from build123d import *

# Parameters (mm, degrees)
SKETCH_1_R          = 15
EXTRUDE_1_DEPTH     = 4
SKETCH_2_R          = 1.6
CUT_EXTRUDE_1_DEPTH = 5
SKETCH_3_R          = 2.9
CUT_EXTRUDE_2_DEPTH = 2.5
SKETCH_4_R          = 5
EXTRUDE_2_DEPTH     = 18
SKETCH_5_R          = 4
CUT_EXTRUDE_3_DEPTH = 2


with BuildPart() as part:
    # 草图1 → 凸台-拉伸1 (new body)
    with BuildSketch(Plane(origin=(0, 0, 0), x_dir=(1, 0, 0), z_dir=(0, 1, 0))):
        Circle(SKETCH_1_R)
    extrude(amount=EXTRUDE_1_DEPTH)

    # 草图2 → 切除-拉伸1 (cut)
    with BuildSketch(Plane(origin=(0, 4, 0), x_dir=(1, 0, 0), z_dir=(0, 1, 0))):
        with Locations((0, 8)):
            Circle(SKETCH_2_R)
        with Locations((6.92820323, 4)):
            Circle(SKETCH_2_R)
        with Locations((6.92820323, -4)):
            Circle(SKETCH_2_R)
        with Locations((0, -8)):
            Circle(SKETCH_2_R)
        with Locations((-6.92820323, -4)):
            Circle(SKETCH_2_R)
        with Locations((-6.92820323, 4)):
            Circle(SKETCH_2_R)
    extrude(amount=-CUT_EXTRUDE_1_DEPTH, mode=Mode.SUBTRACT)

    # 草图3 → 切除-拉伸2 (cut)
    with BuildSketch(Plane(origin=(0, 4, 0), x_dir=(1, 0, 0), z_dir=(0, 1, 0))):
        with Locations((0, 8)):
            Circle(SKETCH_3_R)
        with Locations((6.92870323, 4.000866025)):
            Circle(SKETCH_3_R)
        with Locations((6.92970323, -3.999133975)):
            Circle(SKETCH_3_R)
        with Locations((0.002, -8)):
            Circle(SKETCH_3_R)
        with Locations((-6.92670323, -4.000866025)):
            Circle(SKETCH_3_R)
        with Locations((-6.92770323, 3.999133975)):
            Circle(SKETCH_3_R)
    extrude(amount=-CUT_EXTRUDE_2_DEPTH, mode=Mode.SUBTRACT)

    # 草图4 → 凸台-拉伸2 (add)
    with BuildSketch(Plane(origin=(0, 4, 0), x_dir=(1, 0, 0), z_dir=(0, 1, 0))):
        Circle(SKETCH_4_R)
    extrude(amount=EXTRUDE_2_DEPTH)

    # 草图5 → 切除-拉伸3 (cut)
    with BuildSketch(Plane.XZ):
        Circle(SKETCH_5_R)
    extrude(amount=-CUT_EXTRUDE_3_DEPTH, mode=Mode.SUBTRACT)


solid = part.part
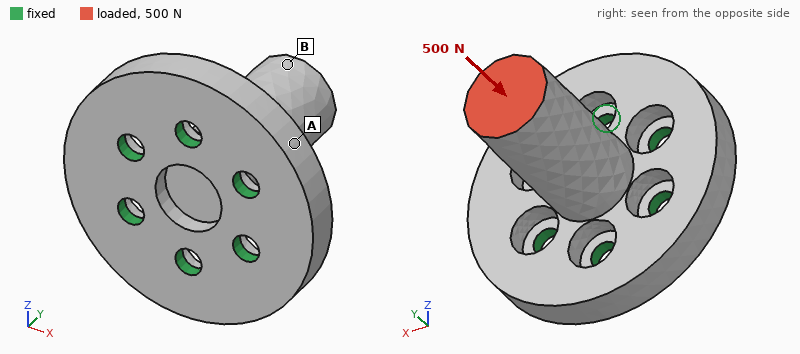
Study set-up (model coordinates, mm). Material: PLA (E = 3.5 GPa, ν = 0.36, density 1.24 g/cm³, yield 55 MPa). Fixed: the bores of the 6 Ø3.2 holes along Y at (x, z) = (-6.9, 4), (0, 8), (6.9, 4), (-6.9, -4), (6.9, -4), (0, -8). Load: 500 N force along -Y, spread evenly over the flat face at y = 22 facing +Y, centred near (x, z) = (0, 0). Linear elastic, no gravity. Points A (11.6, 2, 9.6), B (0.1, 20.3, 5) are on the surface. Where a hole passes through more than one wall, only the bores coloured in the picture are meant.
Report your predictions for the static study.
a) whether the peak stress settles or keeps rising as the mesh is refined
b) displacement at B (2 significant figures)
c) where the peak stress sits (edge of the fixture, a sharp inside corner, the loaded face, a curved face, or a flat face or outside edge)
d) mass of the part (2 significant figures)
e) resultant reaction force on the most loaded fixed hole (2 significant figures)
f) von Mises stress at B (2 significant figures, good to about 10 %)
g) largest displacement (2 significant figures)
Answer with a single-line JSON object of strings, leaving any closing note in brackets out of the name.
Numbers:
{"whether the peak stress settles or keeps rising as the mesh is refined": "keeps rising", "displacement at B": "56 µm", "where the peak stress sits": "edge of the fixture", "mass of the part": "4.6 g", "resultant reaction force on the most loaded fixed hole": "110 N", "von Mises stress at B": "6.4 MPa", "largest displacement": "60 µm"}
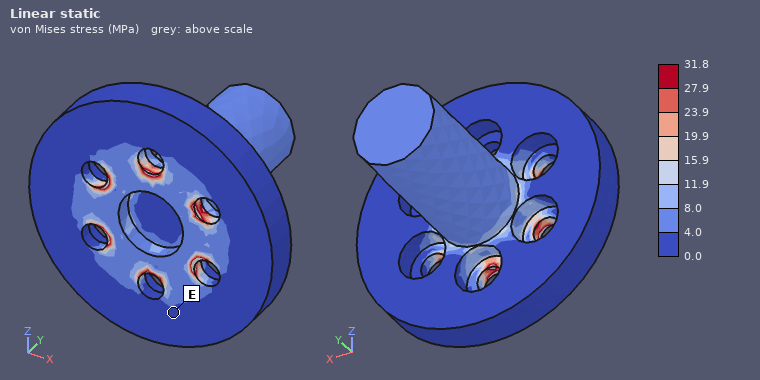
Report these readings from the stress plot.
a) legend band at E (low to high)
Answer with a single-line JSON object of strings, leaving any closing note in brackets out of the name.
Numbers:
{"legend band at E": "0.0 to 4.0 MPa"}
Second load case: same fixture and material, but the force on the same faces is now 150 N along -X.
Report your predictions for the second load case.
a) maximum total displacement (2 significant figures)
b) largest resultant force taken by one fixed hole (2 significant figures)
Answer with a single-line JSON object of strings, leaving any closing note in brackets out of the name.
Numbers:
{"maximum total displacement": "0.40 mm", "largest resultant force taken by one fixed hole": "140 N"}
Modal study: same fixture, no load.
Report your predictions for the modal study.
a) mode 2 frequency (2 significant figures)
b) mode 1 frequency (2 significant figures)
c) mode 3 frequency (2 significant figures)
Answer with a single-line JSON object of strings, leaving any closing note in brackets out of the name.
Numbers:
{"mode 2 frequency": "4200 Hz", "mode 1 frequency": "4200 Hz", "mode 3 frequency": "11 kHz"}
